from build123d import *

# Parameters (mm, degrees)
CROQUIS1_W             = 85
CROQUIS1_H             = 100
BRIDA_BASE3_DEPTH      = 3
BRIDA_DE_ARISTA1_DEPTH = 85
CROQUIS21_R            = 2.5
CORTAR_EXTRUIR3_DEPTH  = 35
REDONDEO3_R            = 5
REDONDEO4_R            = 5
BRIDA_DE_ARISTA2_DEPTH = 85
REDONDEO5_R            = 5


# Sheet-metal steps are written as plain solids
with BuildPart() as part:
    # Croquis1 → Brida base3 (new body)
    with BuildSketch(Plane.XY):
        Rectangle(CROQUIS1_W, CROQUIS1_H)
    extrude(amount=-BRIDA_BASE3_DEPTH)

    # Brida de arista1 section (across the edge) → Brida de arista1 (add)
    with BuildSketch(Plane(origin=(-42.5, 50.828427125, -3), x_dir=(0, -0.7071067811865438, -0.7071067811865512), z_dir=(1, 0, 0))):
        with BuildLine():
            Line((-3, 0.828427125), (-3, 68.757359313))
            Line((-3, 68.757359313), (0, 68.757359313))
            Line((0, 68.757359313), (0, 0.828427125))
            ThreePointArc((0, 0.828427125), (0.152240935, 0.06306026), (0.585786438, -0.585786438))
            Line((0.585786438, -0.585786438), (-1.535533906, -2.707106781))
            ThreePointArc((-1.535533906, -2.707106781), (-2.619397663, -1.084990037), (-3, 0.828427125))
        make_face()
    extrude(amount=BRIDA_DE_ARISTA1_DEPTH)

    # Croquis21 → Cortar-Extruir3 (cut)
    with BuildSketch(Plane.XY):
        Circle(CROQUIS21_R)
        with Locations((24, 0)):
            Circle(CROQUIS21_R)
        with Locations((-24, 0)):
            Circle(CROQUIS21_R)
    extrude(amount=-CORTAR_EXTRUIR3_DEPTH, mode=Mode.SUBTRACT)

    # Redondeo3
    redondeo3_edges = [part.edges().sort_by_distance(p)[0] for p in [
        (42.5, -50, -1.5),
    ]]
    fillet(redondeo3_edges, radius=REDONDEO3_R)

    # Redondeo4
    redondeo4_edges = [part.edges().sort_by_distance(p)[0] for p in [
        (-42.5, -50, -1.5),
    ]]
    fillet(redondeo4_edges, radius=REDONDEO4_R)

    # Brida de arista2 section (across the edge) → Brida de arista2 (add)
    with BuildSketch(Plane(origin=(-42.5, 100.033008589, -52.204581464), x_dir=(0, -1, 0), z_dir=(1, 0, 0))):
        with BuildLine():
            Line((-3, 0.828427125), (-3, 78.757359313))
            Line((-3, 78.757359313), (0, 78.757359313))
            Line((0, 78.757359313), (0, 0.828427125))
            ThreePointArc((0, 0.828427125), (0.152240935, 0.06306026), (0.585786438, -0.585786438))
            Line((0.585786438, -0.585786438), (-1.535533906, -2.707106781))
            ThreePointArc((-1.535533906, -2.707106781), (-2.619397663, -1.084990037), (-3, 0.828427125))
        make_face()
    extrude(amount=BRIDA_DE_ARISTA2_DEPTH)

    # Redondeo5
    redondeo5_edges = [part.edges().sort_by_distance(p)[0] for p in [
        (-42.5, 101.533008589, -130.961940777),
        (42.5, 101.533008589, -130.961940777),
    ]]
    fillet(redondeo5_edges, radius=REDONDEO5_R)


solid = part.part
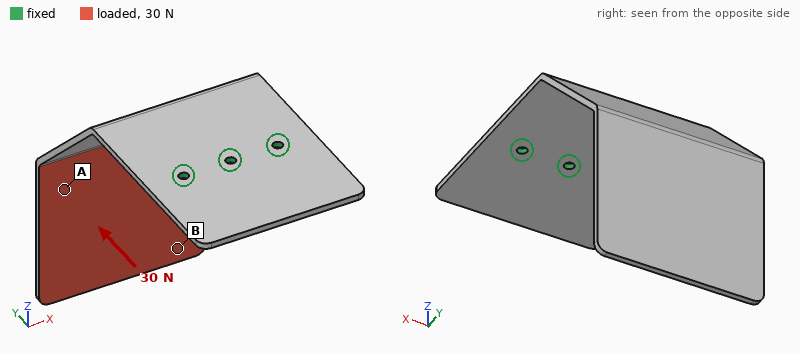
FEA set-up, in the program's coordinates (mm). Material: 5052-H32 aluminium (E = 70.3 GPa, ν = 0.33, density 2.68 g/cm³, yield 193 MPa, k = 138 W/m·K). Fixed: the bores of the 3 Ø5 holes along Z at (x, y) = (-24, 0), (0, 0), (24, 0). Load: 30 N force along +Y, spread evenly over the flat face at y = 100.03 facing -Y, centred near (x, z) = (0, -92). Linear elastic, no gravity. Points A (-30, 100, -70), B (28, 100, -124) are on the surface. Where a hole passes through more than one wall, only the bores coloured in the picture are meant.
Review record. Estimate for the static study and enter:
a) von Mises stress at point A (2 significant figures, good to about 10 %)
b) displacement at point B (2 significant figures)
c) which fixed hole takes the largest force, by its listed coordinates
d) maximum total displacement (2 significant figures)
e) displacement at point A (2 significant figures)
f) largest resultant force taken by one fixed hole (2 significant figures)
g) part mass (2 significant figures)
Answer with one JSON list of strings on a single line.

["5.0 MPa", "2.4 mm", "(0, 0)", "2.6 mm", "1.5 mm", "18 N", "170 g"]
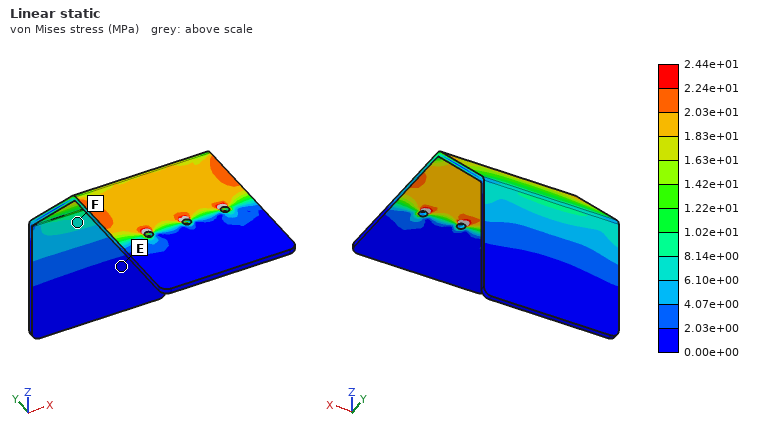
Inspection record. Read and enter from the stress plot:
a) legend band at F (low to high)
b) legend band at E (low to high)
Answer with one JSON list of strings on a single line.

["6.10e+00 to 8.14e+00 MPa", "0.00e+00 to 2.03e+00 MPa"]
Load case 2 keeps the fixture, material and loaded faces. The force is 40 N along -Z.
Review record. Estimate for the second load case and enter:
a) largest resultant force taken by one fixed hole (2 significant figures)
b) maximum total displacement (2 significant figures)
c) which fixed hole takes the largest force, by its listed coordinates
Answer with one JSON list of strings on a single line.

["24 N", "2.1 mm", "(0, 0)"]
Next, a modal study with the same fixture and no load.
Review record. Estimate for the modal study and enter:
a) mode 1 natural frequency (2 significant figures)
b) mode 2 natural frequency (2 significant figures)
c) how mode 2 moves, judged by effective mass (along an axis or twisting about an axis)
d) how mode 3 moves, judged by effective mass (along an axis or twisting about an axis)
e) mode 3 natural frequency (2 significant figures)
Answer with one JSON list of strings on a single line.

["72 Hz", "150 Hz", "along X", "along Z", "290 Hz"]
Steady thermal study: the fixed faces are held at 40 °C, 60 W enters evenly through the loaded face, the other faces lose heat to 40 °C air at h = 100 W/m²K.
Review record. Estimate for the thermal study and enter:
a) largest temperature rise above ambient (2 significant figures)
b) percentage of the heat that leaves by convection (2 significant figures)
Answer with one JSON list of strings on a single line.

["55 K", "95 %"]
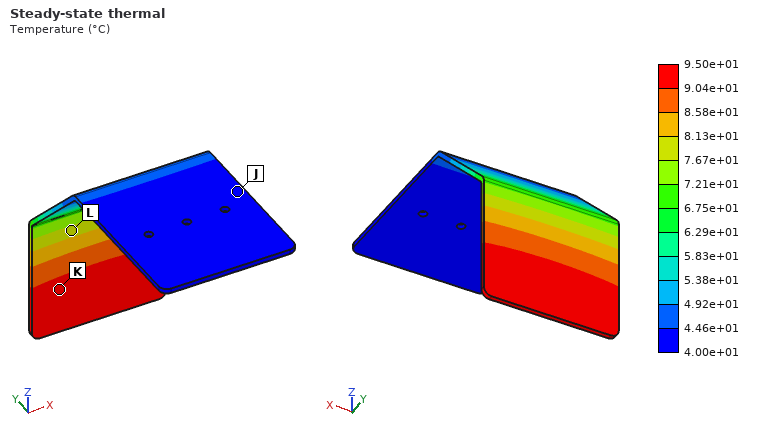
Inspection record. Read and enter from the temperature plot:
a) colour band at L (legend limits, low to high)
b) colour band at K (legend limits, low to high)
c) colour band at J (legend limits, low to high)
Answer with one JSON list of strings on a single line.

["7.67e+01 to 8.13e+01 °C", "9.04e+01 to 9.50e+01 °C", "4.00e+01 to 4.46e+01 °C"]
